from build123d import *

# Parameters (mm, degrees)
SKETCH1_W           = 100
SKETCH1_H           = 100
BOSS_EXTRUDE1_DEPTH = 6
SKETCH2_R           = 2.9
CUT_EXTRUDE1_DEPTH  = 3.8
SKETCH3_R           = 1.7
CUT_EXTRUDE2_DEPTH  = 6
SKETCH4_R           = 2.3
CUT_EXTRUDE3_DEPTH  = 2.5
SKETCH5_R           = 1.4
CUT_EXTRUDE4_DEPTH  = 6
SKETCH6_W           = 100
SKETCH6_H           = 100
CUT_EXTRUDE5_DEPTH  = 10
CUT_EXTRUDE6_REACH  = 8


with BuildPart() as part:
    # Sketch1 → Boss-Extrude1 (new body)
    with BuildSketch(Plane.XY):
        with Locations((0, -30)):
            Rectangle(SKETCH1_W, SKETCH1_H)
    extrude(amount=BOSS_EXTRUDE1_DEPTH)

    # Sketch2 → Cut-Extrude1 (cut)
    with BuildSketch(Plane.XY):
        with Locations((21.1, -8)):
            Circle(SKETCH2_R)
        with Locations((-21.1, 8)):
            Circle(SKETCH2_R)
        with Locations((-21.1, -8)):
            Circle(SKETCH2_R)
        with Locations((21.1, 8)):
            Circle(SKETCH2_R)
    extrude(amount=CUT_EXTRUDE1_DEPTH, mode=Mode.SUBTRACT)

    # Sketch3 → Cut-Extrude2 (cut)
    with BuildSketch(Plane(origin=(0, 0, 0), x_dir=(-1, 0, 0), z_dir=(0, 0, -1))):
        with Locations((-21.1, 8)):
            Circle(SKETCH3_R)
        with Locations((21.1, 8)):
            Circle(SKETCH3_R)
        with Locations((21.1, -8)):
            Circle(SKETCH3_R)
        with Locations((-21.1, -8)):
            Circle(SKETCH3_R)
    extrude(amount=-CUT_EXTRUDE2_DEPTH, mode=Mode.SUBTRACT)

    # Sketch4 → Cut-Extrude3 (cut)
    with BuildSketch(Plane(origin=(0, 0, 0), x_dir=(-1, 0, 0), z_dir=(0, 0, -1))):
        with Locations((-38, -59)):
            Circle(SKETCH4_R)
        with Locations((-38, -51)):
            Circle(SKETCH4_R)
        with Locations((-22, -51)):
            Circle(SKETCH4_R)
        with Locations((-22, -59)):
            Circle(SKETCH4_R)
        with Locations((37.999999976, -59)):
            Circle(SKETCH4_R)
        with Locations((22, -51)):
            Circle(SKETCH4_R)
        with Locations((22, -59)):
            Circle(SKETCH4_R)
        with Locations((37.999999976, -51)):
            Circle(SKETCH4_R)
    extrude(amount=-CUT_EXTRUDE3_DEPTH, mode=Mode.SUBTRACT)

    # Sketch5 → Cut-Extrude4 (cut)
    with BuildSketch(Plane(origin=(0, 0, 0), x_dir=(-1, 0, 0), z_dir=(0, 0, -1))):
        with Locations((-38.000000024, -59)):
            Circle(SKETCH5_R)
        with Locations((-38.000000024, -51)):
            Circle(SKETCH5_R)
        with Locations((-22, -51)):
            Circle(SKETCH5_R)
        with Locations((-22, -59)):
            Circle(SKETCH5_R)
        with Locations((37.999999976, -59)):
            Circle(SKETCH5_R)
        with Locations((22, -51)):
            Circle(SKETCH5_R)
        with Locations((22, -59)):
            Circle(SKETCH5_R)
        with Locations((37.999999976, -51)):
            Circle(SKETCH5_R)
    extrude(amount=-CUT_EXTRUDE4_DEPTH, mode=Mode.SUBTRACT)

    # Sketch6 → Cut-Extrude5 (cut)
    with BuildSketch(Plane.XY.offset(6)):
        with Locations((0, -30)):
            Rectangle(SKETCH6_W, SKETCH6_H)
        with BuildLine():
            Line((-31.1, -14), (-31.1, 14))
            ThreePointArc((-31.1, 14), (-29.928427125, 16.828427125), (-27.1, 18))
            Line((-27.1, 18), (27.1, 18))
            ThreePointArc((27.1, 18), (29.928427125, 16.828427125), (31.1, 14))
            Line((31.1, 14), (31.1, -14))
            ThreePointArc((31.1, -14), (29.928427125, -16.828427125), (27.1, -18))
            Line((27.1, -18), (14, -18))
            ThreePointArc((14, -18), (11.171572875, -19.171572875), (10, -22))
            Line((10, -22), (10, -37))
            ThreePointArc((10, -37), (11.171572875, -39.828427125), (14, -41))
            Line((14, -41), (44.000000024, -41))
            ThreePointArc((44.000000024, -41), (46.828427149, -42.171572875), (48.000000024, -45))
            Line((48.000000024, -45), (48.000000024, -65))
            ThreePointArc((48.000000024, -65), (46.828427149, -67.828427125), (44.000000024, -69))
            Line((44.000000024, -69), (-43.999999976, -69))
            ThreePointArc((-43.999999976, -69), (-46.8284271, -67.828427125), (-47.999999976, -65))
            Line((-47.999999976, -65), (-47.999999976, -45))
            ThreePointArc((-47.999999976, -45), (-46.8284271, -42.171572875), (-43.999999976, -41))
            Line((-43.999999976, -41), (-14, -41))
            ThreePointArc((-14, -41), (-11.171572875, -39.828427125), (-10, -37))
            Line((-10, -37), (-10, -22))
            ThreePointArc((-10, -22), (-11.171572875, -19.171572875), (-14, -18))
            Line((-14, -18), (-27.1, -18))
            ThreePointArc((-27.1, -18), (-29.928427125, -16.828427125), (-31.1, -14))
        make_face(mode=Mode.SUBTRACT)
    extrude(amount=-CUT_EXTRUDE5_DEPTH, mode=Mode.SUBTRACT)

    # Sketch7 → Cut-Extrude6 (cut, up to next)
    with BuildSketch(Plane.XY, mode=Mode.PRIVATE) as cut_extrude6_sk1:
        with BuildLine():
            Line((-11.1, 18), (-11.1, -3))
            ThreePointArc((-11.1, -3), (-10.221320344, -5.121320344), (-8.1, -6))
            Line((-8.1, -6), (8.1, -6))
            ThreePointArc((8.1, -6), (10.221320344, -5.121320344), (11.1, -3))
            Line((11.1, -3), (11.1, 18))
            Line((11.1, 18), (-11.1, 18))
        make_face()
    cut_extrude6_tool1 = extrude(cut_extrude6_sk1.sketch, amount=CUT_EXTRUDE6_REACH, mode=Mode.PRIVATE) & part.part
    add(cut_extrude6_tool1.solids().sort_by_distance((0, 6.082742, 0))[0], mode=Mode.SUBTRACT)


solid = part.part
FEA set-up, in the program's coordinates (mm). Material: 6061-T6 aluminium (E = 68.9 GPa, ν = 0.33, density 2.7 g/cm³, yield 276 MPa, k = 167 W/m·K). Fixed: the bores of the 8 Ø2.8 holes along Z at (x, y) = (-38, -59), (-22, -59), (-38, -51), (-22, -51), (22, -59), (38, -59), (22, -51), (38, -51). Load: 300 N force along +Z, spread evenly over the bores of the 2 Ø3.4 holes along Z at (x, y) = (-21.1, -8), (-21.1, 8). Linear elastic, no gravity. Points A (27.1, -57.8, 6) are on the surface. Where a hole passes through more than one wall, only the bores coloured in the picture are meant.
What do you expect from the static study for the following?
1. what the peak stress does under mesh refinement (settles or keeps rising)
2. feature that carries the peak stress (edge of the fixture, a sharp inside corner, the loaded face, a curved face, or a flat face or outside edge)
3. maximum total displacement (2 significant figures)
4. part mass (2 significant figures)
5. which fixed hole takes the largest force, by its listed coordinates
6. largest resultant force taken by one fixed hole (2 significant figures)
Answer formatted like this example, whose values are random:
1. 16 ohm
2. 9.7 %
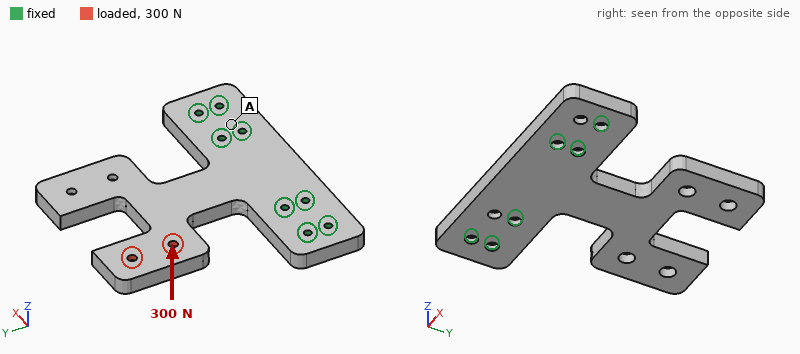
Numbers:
1. keeps rising
2. edge of the fixture
3. 1.2 mm
4. 76 g
5. (-22, -51)
6. 1.1 kN
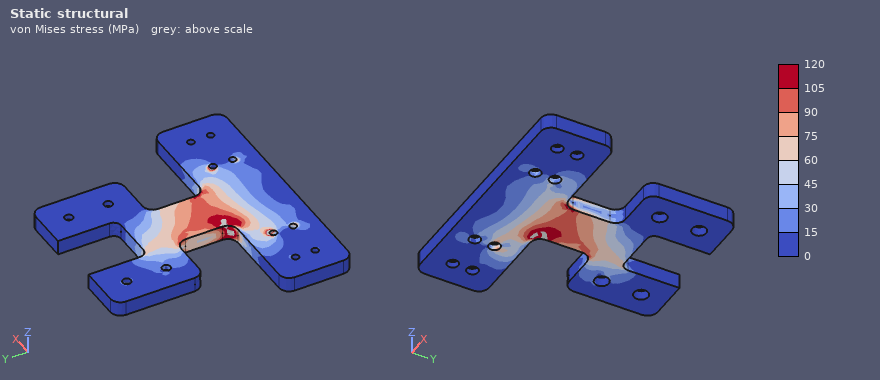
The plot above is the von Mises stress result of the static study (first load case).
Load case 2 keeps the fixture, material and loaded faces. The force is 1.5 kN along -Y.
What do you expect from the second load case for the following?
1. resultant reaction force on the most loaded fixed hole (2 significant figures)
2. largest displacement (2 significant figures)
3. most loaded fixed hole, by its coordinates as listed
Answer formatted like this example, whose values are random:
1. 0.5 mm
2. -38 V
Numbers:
1. 870 N
2. 0.43 mm
3. (-22, -51)
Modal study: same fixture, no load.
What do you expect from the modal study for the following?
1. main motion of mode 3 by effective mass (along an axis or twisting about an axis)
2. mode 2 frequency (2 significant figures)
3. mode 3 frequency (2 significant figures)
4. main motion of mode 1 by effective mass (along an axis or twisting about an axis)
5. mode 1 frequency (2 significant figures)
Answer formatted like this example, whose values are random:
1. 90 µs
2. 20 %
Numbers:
1. along X
2. 1300 Hz
3. 2200 Hz
4. along Z
5. 710 Hz
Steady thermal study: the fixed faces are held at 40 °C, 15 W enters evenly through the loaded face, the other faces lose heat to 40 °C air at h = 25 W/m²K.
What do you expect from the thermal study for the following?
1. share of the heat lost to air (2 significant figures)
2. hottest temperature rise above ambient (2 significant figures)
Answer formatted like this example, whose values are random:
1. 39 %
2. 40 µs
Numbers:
1. 26 %
2. 44 K
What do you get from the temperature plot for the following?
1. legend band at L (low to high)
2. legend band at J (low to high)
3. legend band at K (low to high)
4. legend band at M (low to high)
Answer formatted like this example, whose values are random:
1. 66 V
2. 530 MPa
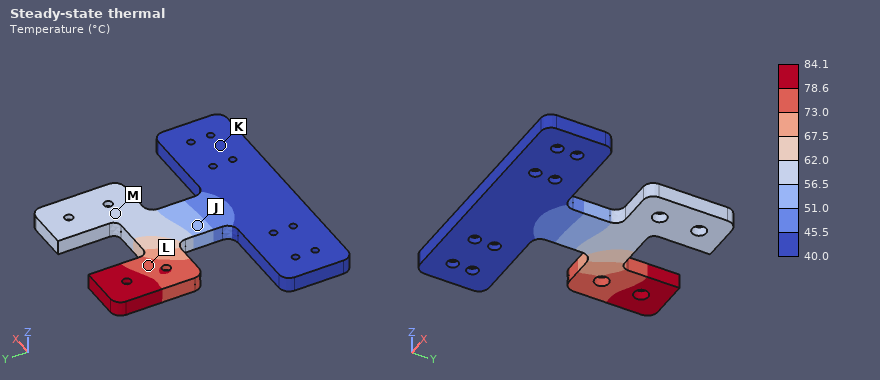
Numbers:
1. 73.0 to 78.6 °C
2. 51.0 to 56.5 °C
3. 40.0 to 45.5 °C
4. 56.5 to 62.0 °C
